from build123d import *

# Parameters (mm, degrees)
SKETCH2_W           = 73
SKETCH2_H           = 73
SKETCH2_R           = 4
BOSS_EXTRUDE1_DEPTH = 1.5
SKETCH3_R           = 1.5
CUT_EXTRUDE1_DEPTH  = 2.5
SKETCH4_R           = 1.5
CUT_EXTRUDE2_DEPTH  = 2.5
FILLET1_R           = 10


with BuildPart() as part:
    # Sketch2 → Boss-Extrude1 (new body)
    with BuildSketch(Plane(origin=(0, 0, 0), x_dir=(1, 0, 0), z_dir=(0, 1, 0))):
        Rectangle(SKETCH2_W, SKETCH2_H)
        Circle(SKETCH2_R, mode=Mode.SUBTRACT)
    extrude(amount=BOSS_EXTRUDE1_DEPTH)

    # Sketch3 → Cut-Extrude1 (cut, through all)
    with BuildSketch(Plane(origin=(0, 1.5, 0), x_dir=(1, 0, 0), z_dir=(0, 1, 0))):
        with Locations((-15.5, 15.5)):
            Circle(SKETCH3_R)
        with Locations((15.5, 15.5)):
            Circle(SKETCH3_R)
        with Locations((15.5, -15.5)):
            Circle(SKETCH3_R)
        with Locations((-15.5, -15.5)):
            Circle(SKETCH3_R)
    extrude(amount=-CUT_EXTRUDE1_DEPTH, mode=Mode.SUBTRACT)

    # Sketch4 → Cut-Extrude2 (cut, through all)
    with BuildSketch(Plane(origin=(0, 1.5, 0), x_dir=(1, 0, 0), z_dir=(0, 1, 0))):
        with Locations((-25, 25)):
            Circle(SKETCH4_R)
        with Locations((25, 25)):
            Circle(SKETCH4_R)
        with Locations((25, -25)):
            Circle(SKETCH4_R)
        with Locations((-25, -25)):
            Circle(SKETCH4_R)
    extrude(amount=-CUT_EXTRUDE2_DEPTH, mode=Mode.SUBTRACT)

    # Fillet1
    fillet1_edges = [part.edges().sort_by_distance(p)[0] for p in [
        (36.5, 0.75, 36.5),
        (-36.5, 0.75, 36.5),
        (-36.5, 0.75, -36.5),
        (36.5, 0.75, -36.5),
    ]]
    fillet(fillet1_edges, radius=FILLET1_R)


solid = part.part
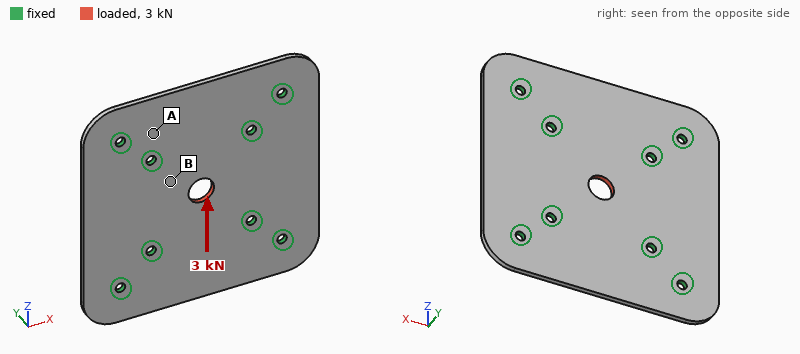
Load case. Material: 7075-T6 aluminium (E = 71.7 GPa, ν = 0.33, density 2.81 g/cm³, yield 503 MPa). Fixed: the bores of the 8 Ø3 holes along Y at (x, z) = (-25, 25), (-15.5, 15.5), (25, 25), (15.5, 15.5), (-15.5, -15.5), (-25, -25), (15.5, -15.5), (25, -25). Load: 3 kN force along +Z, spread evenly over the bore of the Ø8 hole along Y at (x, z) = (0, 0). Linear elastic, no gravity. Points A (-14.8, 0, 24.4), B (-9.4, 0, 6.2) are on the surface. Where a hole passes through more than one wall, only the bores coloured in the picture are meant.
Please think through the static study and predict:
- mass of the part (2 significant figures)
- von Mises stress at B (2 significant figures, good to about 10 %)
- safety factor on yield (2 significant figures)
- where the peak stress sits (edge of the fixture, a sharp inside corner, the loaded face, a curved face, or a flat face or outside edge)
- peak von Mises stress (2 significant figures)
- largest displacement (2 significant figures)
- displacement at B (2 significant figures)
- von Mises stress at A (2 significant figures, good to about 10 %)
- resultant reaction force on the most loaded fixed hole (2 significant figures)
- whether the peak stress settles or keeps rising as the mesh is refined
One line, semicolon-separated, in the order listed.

22 g; 40 MPa; 3.6; the loaded face; 140 MPa; 16 µm; 6.5 µm; 16 MPa; 650 N; settles
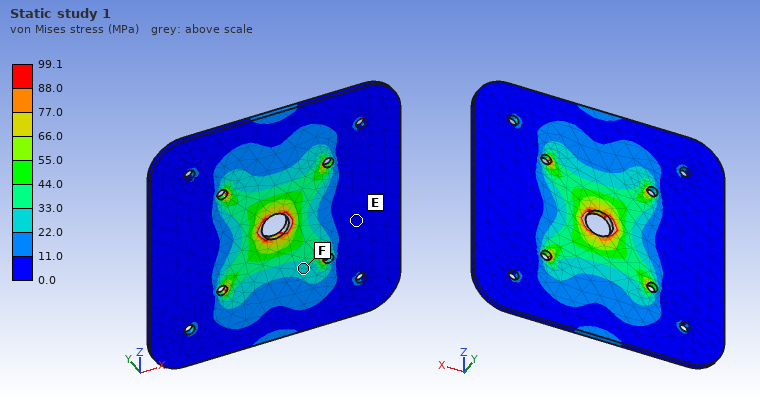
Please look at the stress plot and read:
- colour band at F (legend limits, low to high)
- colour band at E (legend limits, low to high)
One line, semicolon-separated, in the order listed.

22.0 to 33.0 MPa; 0.0 to 11.0 MPa
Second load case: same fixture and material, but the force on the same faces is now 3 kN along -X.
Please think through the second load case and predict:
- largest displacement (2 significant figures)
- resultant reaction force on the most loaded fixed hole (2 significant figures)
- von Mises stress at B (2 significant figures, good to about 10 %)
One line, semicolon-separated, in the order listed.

16 µm; 650 N; 44 MPa
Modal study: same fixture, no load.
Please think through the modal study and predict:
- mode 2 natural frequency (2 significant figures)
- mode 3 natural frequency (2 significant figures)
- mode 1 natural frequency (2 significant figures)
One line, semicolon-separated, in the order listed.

4000 Hz; 4000 Hz; 3800 Hz
